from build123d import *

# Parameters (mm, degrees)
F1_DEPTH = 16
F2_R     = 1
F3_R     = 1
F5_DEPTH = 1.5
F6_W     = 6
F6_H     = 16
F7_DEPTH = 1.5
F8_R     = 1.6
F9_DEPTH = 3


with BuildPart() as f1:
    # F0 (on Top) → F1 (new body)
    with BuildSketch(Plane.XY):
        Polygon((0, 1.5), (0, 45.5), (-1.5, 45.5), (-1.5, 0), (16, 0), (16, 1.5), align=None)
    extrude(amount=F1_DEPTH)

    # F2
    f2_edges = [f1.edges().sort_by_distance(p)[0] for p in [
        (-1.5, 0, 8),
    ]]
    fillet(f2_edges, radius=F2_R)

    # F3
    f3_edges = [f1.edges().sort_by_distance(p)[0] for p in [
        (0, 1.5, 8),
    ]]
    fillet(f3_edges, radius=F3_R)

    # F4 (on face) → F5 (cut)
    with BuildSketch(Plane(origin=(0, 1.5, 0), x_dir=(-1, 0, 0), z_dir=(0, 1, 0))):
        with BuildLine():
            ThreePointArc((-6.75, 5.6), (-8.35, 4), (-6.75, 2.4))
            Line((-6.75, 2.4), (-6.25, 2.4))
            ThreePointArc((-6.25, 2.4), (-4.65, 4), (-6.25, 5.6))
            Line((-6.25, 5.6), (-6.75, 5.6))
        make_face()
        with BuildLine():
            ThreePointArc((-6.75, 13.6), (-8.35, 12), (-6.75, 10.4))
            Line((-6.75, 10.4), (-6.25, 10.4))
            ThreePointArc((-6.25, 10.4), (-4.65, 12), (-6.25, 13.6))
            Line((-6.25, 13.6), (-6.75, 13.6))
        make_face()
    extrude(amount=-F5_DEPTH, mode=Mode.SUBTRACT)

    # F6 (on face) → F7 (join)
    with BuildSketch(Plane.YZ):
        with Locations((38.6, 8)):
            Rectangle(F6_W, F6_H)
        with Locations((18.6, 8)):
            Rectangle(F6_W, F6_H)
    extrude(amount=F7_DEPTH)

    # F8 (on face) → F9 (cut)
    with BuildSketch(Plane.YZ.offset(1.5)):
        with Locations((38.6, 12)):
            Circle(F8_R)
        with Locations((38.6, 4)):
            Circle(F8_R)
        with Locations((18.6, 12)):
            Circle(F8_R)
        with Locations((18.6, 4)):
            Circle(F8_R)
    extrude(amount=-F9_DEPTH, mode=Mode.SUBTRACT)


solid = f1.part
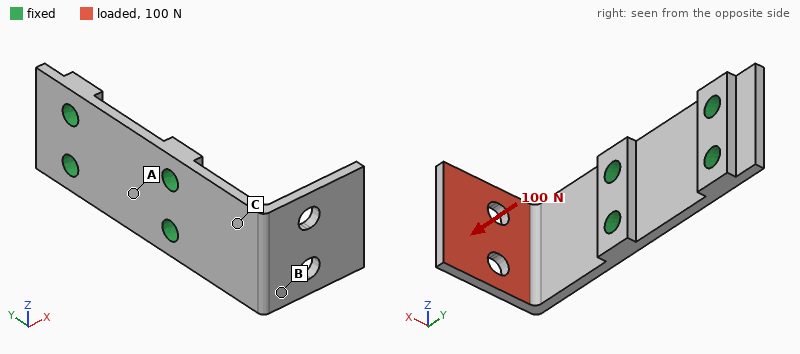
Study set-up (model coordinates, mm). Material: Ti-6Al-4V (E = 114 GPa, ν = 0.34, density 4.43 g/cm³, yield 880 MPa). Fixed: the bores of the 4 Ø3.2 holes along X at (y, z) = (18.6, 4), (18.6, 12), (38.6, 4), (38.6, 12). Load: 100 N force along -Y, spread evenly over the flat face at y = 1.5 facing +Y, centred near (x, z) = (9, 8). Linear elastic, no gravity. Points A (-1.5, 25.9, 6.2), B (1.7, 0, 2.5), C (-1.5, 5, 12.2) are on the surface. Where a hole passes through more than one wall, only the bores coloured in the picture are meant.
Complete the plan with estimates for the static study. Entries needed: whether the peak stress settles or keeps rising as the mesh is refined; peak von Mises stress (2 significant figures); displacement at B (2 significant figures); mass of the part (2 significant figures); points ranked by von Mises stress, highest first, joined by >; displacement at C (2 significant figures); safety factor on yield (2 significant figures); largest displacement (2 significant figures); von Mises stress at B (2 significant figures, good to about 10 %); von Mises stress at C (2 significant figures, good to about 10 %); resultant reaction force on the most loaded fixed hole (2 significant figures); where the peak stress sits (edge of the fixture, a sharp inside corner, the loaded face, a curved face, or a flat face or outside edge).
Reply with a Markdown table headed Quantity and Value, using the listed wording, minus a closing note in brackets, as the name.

| Quantity | Value |
|---|---|
| whether the peak stress settles or keeps rising as the mesh is refined | settles |
| peak von Mises stress | 190 MPa |
| displacement at B | 0.24 mm |
| mass of the part | 7.3 g |
| points ranked by von Mises stress, highest first, joined by > | C > B > A |
| displacement at C | 0.11 mm |
| safety factor on yield | 4.7 |
| largest displacement | 0.60 mm |
| von Mises stress at B | 100 MPa |
| von Mises stress at C | 140 MPa |
| resultant reaction force on the most loaded fixed hole | 52 N |
| where the peak stress sits | a curved face |
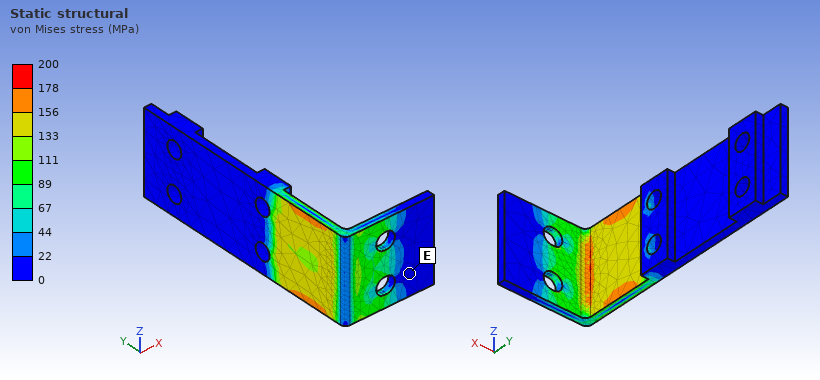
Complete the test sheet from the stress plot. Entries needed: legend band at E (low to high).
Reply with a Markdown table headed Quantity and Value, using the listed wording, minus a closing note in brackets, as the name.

| Quantity | Value |
|---|---|
| legend band at E | 0 to 22 MPa |
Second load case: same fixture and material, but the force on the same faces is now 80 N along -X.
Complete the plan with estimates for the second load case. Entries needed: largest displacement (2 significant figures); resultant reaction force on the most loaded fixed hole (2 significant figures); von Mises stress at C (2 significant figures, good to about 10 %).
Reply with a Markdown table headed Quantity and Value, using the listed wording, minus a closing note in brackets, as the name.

| Quantity | Value |
|---|---|
| largest displacement | 0.32 mm |
| resultant reaction force on the most loaded fixed hole | 41 N |
| von Mises stress at C | 45 MPa |
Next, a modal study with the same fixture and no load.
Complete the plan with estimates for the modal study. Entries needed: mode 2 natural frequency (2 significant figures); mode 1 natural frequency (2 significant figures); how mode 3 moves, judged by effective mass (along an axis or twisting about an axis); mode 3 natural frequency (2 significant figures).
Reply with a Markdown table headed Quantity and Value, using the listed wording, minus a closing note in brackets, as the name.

| Quantity | Value |
|---|---|
| mode 2 natural frequency | 3000 Hz |
| mode 1 natural frequency | 1700 Hz |
| how mode 3 moves, judged by effective mass | along X |
| mode 3 natural frequency | 4600 Hz |
